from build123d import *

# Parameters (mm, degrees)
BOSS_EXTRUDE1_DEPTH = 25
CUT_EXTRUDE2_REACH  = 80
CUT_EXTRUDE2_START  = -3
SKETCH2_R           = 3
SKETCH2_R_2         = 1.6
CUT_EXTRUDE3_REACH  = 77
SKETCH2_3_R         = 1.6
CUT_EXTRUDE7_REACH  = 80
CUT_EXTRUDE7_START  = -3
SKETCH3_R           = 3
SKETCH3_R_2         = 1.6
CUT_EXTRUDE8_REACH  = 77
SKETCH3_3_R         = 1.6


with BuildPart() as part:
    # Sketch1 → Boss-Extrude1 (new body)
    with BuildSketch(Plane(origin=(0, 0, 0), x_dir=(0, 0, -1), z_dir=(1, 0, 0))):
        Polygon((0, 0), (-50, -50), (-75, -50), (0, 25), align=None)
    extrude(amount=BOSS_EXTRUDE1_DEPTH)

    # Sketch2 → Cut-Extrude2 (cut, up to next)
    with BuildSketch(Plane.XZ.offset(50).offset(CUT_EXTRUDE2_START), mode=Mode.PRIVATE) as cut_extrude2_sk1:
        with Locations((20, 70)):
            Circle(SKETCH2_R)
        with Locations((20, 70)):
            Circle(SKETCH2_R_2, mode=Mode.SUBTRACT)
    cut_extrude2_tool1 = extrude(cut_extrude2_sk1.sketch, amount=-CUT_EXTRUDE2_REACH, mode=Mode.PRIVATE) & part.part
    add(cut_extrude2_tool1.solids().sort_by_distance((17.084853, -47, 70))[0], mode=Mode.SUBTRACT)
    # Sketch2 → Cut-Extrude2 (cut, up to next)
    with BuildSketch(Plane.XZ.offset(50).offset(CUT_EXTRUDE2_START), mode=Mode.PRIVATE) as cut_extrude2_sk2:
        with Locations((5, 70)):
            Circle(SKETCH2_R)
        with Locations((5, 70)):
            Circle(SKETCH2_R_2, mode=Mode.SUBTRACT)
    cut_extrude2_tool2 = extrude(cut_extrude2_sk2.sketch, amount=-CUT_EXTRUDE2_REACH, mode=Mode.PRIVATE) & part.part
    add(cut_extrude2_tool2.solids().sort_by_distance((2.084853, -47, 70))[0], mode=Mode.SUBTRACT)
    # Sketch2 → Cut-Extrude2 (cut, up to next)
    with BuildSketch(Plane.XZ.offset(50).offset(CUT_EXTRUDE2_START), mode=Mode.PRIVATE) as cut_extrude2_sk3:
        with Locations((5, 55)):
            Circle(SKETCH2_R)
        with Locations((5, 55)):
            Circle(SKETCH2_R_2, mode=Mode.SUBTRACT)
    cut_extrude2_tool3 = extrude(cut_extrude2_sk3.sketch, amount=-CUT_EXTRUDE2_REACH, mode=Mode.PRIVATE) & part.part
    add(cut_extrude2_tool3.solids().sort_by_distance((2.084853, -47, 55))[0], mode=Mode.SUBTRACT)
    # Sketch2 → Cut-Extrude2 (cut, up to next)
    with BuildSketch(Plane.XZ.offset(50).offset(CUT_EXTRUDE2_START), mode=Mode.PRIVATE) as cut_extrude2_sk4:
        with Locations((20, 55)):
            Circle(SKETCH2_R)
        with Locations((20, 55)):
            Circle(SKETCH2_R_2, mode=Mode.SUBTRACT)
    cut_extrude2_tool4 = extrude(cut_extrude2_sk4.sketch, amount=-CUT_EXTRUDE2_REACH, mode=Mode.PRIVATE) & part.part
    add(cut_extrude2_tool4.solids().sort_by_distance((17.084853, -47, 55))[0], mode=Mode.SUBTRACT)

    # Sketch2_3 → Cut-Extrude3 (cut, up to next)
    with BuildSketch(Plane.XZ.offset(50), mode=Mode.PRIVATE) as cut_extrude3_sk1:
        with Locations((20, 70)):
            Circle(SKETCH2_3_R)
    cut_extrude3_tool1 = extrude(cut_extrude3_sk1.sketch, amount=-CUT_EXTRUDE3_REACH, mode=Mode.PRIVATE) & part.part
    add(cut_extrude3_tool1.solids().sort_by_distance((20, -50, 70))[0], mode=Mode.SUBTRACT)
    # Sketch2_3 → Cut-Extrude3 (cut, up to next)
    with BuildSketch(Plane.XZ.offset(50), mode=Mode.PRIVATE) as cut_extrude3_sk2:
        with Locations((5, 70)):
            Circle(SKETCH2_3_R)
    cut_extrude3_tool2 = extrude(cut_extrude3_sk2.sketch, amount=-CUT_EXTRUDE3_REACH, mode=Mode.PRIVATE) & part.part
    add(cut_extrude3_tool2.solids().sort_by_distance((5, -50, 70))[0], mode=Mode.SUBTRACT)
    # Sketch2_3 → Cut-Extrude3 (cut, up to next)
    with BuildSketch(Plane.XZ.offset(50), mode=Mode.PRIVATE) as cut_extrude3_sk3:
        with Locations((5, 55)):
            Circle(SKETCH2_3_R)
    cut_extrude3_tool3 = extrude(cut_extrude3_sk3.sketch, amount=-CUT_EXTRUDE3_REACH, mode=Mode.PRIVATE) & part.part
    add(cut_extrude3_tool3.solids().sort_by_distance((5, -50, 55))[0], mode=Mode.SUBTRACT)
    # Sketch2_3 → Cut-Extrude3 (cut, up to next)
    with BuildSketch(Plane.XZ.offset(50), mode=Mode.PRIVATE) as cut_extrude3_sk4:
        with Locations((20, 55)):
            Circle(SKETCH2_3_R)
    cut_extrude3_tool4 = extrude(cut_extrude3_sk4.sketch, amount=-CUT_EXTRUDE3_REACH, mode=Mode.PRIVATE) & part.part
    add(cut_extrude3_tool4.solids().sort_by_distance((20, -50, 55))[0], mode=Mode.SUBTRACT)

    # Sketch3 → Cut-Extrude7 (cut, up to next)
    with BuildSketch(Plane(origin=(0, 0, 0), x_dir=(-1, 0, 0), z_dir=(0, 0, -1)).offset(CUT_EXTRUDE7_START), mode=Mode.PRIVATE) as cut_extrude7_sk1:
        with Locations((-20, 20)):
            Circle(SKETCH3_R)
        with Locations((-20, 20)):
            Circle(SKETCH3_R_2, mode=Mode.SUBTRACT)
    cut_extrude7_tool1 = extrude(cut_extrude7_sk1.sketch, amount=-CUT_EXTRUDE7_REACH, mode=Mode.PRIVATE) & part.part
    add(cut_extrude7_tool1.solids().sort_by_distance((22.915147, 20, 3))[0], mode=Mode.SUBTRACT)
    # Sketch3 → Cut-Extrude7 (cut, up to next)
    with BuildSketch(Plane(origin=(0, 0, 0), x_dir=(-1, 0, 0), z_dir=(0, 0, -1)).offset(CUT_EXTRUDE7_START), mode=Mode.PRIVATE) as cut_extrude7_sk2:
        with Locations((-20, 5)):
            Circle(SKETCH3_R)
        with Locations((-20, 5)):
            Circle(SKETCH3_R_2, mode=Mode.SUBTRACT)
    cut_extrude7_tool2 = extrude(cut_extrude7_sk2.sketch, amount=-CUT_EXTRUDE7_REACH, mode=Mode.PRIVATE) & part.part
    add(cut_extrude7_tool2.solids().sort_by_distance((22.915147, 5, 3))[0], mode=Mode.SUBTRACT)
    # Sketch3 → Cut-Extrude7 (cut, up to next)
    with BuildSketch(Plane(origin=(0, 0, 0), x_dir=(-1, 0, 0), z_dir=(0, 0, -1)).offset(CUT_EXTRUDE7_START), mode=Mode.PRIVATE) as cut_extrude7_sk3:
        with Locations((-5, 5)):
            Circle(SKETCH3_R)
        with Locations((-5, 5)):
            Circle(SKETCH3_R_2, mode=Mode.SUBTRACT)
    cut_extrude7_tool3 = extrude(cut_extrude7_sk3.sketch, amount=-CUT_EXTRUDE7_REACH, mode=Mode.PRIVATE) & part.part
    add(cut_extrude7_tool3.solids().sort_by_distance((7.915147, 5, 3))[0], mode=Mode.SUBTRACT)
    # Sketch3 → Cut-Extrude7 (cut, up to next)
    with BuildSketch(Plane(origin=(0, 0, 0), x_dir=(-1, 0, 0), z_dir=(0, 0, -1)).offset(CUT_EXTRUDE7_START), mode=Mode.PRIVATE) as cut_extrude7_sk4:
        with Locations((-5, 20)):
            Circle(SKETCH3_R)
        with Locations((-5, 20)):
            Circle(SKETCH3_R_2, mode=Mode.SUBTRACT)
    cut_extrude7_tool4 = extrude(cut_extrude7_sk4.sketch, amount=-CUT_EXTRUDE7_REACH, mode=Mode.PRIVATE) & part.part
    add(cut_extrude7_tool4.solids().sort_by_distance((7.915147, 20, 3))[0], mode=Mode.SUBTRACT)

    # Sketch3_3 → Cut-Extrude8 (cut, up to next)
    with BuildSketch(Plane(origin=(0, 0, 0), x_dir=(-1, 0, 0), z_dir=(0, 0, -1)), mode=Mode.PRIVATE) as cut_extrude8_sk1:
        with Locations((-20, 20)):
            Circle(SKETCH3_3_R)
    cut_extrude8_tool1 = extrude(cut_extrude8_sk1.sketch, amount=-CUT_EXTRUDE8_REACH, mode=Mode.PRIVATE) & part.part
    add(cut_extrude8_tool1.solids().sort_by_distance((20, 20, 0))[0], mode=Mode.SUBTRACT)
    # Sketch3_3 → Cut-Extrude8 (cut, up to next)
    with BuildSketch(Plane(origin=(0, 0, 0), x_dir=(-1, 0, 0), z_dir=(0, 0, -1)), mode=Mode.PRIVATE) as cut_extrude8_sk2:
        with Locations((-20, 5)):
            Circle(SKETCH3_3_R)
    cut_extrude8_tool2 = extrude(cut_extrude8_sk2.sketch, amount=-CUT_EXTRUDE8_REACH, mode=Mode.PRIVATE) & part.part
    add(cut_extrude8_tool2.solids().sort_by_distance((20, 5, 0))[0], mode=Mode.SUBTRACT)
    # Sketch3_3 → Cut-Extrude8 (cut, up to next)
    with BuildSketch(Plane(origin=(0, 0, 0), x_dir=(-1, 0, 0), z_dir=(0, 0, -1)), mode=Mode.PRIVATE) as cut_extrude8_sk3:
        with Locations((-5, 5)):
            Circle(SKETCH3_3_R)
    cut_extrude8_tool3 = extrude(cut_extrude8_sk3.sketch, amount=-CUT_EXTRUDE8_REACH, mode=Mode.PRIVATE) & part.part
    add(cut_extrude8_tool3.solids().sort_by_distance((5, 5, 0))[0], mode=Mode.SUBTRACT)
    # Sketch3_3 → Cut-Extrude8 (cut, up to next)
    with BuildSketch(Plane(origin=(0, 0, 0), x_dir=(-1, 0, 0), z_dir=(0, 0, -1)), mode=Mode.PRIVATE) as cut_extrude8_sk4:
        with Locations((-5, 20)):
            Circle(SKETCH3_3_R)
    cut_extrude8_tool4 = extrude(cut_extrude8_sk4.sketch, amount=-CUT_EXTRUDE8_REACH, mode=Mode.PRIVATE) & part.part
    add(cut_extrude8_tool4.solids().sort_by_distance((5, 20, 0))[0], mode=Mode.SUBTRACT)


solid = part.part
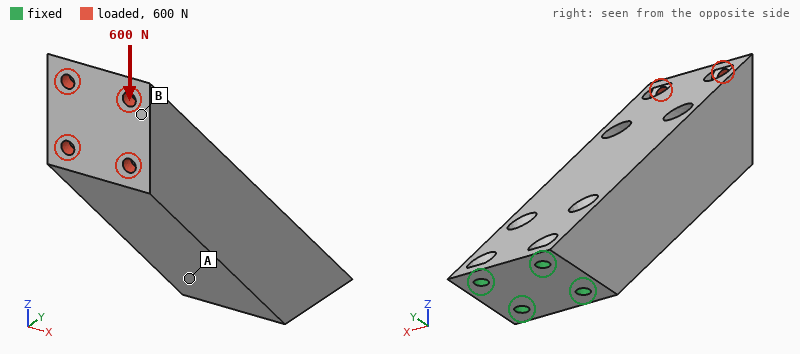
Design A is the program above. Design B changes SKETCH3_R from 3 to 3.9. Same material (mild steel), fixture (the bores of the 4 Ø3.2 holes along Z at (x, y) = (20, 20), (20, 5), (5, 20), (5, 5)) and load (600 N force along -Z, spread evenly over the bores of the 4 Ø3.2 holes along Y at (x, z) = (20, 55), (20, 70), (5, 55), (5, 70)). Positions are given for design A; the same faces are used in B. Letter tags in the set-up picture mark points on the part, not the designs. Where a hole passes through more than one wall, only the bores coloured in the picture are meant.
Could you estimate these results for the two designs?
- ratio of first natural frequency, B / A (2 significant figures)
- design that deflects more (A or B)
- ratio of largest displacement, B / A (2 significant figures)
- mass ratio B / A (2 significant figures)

0.91
B
1.2
0.98
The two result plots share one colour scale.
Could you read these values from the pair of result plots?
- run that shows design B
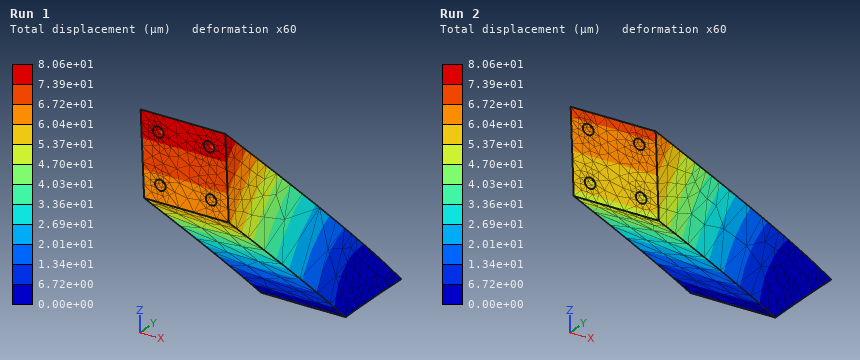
Run 1
